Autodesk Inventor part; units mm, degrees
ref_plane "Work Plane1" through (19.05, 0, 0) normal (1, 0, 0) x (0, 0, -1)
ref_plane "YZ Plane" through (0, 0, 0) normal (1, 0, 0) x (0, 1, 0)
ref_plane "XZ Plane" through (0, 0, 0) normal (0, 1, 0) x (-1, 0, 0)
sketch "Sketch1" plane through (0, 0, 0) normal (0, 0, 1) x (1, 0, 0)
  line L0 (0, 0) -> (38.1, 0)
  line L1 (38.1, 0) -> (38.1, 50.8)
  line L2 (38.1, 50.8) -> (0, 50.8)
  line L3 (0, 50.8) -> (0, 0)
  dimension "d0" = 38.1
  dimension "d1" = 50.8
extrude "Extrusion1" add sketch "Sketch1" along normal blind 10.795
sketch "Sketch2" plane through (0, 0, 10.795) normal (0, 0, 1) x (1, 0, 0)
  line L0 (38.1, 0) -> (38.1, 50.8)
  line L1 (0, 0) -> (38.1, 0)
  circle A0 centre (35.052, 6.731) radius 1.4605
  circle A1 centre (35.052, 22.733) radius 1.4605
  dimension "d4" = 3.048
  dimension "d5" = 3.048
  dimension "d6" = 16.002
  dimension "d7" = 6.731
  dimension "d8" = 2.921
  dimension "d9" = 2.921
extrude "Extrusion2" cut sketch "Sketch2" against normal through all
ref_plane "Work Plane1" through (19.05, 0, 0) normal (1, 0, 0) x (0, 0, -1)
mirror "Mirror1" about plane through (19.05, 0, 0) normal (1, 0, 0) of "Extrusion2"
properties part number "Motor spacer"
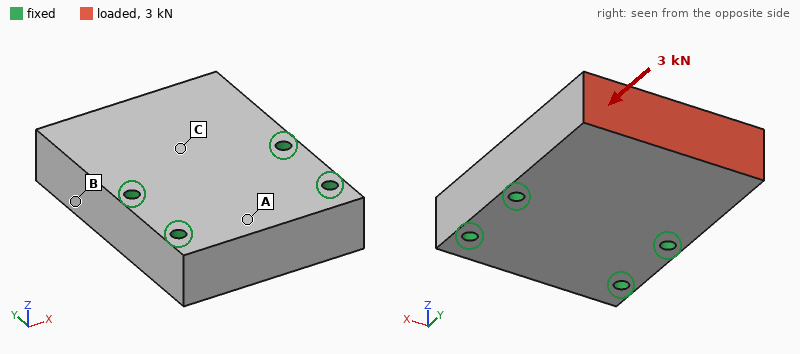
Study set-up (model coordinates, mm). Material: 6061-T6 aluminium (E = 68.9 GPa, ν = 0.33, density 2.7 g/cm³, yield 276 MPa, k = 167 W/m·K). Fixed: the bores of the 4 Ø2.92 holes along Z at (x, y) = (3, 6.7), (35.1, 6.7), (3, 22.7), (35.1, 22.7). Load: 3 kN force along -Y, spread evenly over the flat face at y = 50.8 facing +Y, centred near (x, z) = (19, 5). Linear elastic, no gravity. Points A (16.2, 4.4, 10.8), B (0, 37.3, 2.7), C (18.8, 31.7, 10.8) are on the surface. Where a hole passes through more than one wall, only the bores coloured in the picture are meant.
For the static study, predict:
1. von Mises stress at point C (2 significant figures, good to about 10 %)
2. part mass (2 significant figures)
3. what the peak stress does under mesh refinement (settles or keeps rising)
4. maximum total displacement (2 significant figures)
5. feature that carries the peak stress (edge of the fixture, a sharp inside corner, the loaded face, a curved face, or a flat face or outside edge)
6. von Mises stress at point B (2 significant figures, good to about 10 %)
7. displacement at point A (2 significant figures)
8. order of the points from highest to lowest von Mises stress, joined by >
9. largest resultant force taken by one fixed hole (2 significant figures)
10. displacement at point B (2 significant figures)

4.7 MPa
56 g
keeps rising
3.6 µm
edge of the fixture
8.3 MPa
0.85 µm
B > C > A
1.2 kN
2.2 µm
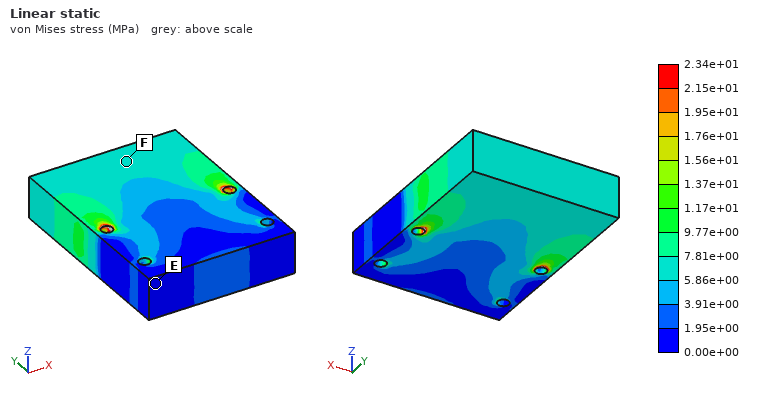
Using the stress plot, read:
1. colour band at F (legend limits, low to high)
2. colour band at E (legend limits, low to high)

5.86e+00 to 7.81e+00 MPa
0.00e+00 to 1.95e+00 MPa
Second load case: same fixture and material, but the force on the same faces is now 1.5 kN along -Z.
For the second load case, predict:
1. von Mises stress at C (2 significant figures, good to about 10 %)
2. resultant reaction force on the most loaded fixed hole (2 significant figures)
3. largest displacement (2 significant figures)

32 MPa
1.2 kN
61 µm
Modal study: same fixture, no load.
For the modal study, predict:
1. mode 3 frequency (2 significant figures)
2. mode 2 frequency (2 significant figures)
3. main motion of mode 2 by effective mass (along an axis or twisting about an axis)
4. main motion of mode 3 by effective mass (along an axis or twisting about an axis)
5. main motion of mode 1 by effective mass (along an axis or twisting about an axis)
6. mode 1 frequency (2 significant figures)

20 kHz
17 kHz
twisting about Y
along X
along Z
8400 Hz
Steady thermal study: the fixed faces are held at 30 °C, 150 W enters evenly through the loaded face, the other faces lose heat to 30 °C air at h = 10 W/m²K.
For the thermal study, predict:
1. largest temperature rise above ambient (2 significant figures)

69 K
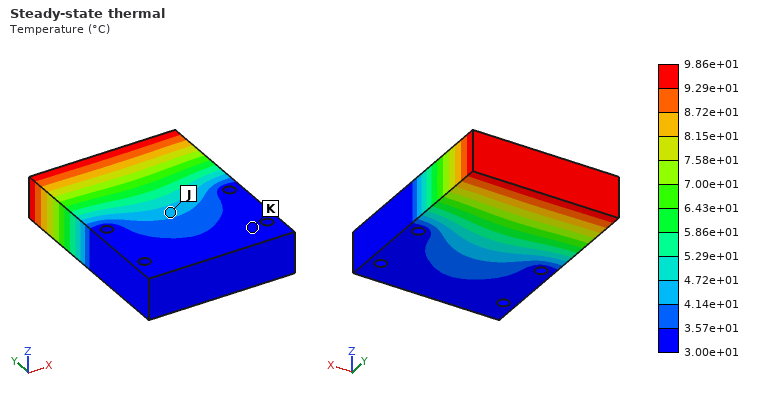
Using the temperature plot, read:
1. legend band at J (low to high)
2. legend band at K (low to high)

4.14e+01 to 4.72e+01 °C
3.00e+01 to 3.57e+01 °C
